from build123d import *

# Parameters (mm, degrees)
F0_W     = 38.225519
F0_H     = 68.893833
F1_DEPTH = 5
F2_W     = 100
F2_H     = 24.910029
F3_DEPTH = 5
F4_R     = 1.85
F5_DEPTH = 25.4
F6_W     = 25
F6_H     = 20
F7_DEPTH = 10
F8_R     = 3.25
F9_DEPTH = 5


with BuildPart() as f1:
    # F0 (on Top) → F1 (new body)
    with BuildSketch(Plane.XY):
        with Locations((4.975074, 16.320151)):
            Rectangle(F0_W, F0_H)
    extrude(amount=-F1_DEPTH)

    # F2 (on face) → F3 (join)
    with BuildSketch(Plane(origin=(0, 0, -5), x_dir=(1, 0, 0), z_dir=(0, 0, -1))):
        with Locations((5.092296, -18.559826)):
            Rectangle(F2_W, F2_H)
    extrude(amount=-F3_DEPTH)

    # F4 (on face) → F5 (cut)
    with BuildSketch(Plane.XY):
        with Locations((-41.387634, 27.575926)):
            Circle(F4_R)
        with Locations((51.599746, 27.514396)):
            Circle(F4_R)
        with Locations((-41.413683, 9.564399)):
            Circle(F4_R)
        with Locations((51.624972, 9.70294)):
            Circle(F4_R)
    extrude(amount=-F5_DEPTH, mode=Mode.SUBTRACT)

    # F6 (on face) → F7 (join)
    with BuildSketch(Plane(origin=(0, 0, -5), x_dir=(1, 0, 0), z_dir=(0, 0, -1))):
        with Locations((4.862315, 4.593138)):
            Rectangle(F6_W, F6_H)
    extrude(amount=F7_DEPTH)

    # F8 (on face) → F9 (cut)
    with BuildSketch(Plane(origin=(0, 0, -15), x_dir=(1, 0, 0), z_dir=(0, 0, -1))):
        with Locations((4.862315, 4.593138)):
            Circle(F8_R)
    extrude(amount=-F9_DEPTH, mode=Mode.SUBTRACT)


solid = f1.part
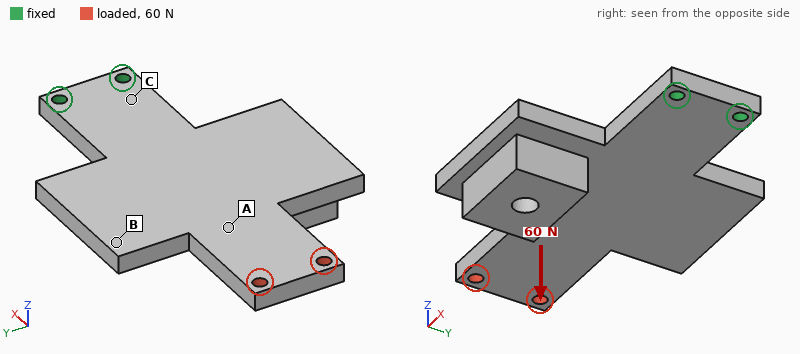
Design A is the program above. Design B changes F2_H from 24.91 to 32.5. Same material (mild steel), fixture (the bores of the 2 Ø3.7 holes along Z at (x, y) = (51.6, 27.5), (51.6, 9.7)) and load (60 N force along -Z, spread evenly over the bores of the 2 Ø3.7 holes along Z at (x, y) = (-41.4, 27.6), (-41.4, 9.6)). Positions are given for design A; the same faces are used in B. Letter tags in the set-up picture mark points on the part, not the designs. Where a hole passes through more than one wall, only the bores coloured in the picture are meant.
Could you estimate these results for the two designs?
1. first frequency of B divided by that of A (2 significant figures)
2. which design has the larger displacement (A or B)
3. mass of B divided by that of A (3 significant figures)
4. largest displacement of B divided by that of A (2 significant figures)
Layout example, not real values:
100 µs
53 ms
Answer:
1.1
A
1.09
0.78
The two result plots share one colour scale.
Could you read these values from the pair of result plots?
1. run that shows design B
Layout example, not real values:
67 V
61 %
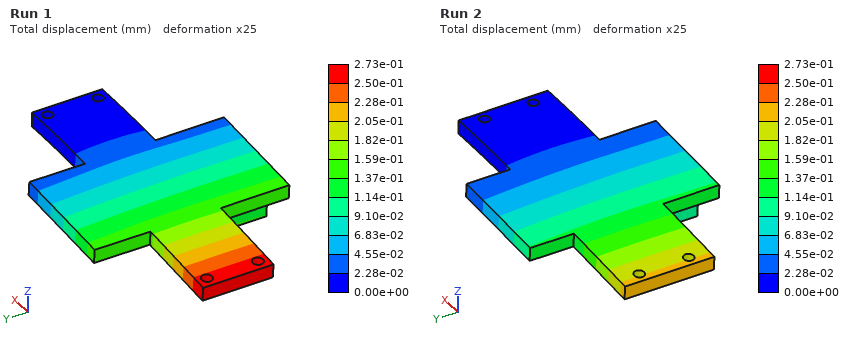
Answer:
Run 2
